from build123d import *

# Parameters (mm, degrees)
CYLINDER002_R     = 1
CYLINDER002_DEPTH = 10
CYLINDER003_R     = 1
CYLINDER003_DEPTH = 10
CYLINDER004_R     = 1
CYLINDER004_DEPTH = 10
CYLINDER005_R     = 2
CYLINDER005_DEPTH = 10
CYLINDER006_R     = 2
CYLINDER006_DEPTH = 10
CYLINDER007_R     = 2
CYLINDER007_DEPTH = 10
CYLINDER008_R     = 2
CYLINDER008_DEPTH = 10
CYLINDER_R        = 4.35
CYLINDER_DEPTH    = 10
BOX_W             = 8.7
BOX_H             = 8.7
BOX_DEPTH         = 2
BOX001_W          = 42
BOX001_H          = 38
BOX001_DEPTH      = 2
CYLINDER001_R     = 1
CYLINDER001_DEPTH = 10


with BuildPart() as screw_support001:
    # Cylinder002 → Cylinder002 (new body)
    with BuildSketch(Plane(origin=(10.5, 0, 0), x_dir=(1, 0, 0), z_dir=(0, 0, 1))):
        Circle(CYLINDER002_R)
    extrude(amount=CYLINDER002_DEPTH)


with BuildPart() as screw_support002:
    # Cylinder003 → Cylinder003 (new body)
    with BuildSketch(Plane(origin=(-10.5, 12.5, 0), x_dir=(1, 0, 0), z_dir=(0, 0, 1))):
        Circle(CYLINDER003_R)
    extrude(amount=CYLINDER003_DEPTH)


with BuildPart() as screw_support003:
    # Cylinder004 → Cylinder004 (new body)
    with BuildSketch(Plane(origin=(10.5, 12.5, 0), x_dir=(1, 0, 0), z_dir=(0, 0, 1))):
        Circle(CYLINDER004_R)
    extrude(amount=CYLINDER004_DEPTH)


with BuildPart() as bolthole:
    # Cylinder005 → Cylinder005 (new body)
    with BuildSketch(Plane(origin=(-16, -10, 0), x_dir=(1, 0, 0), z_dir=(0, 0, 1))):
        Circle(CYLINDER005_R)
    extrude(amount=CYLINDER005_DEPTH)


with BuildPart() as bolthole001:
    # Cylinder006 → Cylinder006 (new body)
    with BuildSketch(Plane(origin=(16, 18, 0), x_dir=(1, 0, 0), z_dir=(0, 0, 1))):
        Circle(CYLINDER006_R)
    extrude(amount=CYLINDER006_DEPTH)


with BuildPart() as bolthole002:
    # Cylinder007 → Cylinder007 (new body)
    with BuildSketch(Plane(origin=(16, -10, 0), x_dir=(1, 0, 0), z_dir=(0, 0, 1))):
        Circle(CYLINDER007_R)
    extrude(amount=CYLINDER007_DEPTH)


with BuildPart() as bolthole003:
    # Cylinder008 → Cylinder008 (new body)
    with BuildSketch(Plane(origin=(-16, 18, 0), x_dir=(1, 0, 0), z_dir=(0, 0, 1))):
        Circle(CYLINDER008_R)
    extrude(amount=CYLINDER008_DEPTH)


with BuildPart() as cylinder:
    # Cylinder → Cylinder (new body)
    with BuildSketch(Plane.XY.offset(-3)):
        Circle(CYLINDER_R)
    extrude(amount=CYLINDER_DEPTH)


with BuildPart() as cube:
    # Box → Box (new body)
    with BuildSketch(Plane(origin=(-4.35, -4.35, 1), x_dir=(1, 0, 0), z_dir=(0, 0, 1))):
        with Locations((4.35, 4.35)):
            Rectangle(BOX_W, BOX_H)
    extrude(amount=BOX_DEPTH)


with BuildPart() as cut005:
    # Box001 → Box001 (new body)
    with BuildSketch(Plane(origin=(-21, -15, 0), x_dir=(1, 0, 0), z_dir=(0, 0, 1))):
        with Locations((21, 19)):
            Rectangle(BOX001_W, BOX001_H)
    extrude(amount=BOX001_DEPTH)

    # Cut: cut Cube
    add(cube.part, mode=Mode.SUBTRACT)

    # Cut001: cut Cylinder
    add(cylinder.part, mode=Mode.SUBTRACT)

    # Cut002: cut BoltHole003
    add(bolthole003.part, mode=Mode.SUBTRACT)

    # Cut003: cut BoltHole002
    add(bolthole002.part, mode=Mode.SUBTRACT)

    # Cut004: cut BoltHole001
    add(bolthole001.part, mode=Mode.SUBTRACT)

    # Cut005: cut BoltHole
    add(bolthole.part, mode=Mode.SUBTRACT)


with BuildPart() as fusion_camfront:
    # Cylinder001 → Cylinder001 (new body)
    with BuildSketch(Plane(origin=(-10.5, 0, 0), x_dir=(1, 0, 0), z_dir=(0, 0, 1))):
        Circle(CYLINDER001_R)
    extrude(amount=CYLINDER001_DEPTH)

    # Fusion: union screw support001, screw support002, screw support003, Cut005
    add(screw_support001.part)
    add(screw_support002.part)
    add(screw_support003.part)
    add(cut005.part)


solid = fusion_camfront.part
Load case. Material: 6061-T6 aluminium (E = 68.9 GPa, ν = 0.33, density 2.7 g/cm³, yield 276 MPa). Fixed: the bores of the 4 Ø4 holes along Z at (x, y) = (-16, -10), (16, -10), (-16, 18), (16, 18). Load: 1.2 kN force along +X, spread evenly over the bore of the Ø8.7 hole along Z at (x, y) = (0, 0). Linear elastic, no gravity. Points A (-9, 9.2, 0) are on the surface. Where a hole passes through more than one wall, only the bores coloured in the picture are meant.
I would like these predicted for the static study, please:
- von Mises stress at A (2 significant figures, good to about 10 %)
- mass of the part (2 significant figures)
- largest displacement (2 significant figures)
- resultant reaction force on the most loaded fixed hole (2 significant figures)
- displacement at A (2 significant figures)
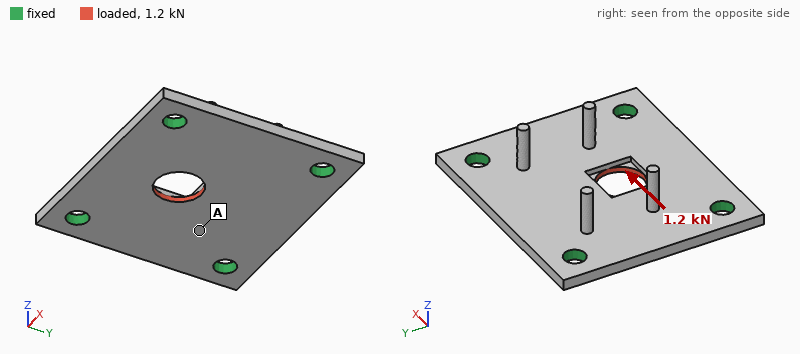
15 MPa
8.3 g
6.6 µm
380 N
2.9 µm
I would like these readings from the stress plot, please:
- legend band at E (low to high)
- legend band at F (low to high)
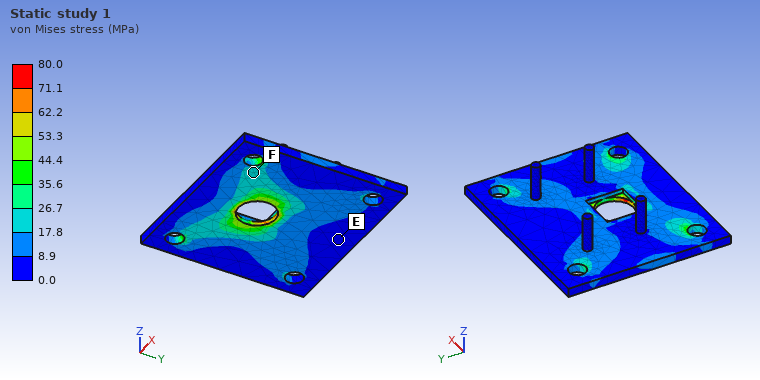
0.0 to 8.9 MPa
17.8 to 26.7 MPa
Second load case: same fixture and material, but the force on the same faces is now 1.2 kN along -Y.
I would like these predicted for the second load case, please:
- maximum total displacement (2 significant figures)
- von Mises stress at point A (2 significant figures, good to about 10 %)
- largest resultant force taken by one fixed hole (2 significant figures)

9.3 µm
19 MPa
350 N
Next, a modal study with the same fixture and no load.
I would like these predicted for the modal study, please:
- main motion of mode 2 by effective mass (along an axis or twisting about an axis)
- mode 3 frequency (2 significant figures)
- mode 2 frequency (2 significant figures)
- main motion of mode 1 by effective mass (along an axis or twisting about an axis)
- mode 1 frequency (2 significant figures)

twisting about X
14 kHz
13 kHz
along Z
8900 Hz
